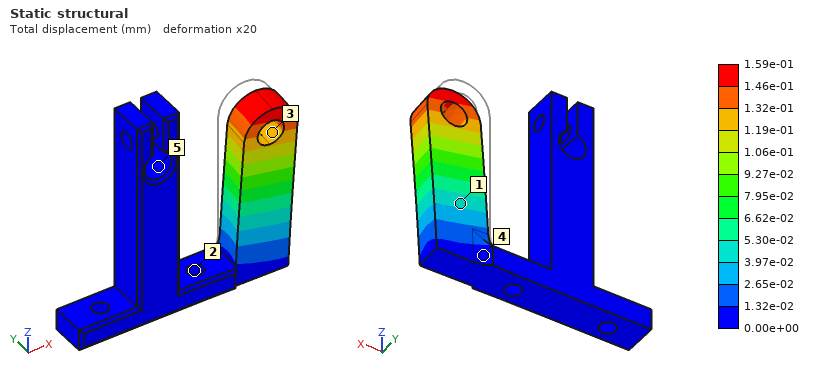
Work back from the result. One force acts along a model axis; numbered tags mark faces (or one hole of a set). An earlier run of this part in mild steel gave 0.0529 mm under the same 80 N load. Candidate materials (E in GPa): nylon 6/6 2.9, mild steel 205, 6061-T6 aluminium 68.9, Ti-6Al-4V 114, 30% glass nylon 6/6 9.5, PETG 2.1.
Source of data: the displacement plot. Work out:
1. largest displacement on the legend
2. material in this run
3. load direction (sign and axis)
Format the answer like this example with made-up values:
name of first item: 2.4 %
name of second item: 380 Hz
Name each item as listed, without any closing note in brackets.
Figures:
largest displacement on the legend: 1.59e-01 mm
material in this run: 6061-T6 aluminium
load direction: -Y
